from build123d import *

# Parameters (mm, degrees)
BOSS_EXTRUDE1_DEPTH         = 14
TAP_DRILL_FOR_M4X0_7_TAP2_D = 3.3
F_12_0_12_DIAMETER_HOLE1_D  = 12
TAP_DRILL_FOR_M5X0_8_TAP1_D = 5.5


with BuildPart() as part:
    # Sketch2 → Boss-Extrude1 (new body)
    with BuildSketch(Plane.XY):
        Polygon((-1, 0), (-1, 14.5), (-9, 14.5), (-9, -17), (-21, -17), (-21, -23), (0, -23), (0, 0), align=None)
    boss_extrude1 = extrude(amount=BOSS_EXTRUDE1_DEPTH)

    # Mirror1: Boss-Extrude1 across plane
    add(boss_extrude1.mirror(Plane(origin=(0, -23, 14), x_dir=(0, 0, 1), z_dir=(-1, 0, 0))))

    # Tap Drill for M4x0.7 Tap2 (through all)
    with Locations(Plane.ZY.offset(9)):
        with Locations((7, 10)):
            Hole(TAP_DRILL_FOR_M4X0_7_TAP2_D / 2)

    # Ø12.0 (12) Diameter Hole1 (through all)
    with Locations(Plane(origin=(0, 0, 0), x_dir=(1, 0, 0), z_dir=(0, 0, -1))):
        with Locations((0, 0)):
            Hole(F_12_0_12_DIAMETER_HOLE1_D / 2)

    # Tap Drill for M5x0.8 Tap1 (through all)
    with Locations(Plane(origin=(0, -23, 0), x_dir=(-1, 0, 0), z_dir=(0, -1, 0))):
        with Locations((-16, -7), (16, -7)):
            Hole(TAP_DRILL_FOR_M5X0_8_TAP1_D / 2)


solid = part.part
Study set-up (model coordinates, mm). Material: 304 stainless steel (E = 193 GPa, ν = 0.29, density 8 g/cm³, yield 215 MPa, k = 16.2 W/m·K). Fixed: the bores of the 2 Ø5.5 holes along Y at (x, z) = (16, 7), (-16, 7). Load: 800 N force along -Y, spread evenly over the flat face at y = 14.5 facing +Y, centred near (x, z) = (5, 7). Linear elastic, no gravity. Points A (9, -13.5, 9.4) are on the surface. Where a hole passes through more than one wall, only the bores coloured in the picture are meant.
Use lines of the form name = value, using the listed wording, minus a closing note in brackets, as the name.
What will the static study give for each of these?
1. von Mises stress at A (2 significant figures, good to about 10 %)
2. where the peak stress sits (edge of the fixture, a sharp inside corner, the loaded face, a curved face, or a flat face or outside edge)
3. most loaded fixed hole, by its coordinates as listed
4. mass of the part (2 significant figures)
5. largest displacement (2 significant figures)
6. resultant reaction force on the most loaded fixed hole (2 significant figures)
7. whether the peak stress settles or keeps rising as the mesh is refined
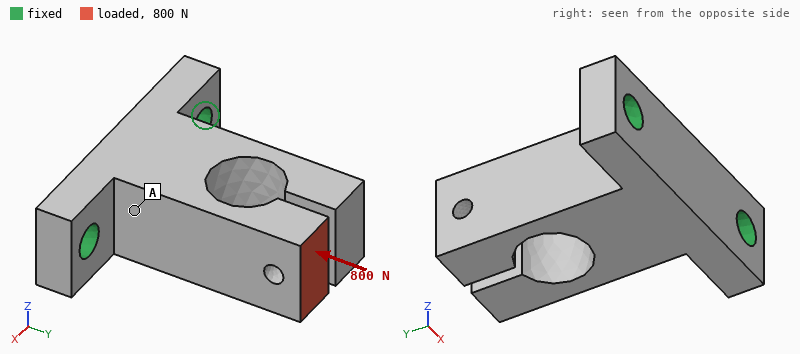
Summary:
von Mises stress at A = 13 MPa
where the peak stress sits = a sharp inside corner
most loaded fixed hole, by its coordinates as listed = (16, 7)
mass of the part = 74 g
largest displacement = 33 µm
resultant reaction force on the most loaded fixed hole = 590 N
whether the peak stress settles or keeps rising as the mesh is refined = keeps rising
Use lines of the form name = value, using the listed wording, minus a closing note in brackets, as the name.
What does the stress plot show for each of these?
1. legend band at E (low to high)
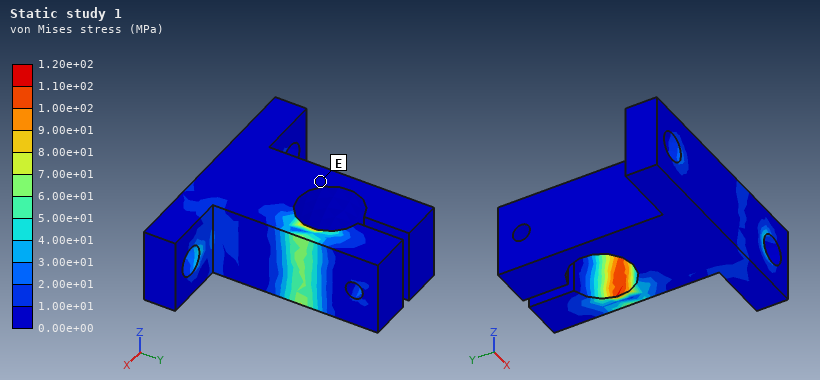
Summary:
legend band at E = 0.00e+00 to 1.00e+01 MPa
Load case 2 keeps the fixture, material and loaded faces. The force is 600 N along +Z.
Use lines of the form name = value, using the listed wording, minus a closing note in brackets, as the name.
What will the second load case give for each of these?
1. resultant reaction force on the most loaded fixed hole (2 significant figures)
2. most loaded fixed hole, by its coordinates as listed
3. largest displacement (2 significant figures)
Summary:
resultant reaction force on the most loaded fixed hole = 390 N
most loaded fixed hole, by its coordinates as listed = (16, 7)
largest displacement = 75 µm
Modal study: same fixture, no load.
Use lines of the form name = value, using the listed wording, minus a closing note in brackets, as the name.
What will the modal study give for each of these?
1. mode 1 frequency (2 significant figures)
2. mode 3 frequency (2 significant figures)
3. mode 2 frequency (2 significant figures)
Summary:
mode 1 frequency = 4200 Hz
mode 3 frequency = 4400 Hz
mode 2 frequency = 4200 Hz
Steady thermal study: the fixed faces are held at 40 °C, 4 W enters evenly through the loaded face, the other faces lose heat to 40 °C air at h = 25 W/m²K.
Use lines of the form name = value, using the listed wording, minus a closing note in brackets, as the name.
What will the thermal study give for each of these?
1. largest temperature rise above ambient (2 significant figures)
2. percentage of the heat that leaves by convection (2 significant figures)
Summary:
largest temperature rise above ambient = 83 K
percentage of the heat that leaves by convection = 45 %
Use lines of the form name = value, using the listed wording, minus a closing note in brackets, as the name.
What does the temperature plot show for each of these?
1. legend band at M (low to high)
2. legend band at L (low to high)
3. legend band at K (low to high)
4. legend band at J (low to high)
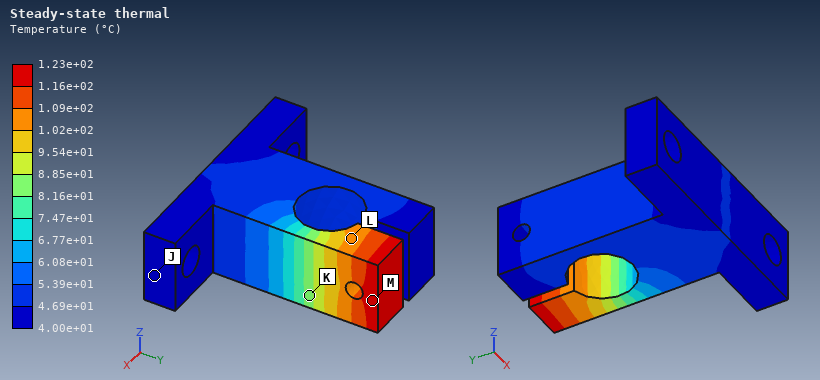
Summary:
legend band at M = 1.16e+02 to 1.23e+02 °C
legend band at L = 1.02e+02 to 1.09e+02 °C
legend band at K = 8.16e+01 to 8.85e+01 °C
legend band at J = 4.00e+01 to 4.69e+01 °C
